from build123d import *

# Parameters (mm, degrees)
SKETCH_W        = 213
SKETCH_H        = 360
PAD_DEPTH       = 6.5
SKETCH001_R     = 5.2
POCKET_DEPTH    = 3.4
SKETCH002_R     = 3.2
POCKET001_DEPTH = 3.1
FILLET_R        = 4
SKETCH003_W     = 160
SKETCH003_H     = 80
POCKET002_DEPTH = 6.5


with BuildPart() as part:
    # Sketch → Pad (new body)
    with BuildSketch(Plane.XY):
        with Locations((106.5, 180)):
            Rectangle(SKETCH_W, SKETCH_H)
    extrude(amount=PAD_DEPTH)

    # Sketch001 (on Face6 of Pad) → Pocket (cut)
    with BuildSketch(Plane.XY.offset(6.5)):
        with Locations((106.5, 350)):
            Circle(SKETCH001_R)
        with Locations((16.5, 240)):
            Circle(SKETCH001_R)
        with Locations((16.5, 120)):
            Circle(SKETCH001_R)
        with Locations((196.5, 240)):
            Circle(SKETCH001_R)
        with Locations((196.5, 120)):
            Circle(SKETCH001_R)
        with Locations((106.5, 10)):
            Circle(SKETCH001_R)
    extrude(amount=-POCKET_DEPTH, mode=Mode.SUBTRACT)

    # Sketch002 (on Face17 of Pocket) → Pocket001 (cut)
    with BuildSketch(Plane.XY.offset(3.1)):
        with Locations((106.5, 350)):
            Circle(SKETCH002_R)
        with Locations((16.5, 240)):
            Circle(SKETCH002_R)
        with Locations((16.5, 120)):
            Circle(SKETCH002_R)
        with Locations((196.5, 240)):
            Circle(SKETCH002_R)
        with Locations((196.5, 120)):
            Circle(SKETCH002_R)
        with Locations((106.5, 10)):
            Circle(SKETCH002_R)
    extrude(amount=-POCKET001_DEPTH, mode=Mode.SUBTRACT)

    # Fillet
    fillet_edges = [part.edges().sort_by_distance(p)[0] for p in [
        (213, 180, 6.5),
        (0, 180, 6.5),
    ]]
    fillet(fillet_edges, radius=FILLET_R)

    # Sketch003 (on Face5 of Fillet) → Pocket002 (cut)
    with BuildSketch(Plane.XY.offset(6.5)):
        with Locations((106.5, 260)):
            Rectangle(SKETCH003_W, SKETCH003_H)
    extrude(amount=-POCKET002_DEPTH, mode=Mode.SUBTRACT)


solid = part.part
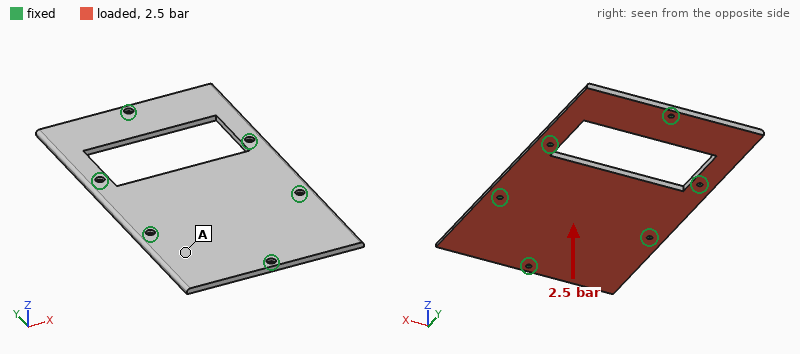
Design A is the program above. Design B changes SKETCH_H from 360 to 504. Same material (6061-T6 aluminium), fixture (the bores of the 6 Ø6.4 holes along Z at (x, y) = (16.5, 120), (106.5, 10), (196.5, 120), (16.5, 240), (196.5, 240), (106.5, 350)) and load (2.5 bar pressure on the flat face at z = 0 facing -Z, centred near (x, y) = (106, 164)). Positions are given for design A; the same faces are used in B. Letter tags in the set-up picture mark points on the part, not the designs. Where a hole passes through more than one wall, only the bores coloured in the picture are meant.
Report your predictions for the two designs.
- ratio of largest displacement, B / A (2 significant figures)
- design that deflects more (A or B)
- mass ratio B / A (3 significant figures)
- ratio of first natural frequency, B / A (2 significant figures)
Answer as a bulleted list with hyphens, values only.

- 3.3
- B
- 1.48
- 0.57
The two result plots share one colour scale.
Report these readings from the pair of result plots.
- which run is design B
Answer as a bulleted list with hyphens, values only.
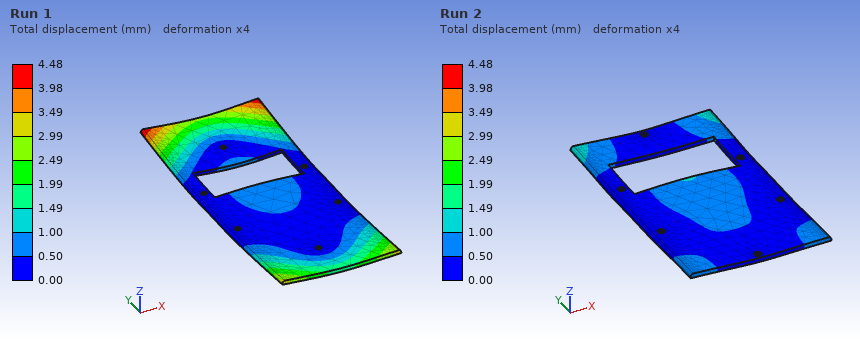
- Run 1
